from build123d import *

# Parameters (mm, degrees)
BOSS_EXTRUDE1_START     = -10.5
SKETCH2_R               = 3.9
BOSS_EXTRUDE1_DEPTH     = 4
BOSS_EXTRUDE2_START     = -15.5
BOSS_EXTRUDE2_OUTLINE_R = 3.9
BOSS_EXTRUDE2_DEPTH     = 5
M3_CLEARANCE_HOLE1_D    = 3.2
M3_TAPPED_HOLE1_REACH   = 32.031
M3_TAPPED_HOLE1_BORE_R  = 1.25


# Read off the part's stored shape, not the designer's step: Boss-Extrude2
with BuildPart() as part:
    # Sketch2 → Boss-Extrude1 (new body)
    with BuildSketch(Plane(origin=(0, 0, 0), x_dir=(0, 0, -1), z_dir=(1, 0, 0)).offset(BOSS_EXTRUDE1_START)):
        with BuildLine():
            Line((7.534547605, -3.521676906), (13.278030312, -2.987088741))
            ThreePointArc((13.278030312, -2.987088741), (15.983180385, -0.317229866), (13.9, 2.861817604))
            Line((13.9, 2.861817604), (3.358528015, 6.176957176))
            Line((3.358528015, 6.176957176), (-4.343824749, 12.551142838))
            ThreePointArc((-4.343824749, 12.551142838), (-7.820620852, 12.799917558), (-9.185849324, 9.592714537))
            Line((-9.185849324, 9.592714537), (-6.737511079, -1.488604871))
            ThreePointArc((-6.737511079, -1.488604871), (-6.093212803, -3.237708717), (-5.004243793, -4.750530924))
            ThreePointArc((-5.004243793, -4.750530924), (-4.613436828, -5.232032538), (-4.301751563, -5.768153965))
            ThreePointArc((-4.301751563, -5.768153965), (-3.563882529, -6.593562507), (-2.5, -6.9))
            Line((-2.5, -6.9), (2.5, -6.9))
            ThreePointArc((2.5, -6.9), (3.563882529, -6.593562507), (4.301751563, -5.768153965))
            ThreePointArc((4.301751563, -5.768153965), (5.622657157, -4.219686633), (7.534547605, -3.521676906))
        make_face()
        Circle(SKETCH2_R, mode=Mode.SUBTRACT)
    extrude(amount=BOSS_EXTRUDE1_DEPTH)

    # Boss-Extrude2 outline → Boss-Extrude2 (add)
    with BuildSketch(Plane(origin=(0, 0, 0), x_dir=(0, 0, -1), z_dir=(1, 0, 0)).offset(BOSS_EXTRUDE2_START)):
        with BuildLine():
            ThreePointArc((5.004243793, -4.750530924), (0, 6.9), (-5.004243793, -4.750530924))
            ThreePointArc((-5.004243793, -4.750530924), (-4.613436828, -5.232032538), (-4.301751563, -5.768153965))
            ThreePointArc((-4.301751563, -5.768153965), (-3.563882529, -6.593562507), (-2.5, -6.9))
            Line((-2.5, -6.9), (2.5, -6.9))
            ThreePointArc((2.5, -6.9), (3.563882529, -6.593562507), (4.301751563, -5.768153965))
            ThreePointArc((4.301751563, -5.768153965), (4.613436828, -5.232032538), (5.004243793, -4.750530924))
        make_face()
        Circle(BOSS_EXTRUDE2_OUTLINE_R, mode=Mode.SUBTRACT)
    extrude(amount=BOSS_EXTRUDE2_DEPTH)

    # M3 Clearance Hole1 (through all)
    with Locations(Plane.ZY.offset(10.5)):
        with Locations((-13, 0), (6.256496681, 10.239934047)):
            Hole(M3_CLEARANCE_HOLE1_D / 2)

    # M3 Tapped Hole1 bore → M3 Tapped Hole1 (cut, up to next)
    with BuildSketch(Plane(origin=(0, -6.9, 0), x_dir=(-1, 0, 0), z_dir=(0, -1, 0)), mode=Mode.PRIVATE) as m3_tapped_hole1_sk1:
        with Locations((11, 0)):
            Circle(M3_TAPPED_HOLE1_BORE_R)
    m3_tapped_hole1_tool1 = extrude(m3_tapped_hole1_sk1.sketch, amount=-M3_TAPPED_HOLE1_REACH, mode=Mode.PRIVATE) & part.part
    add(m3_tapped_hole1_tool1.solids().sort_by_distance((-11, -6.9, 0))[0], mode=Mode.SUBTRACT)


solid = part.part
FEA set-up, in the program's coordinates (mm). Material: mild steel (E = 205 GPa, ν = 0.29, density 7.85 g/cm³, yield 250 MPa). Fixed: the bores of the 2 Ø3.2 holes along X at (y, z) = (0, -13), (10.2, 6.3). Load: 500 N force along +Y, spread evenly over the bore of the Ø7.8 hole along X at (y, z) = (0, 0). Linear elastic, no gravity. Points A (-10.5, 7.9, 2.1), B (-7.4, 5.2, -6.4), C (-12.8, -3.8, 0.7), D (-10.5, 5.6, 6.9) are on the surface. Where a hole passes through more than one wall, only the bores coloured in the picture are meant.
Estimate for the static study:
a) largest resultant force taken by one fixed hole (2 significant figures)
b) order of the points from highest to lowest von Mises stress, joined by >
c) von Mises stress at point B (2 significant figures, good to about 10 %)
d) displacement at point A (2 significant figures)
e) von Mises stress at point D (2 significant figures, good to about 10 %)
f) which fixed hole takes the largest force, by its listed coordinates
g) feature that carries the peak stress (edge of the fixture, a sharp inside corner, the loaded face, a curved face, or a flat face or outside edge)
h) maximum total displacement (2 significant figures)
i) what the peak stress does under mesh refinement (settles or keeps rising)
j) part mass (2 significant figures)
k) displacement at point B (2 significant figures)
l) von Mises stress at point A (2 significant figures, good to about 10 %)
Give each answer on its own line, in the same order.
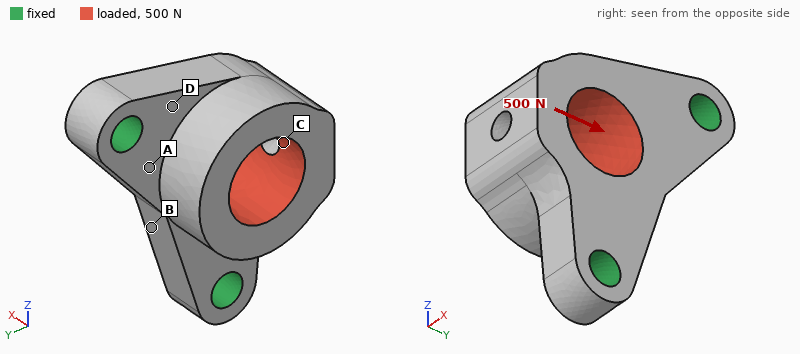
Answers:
370 N
D > A > B > C
11 MPa
0.95 µm
37 MPa
(10.2, 6.3)
edge of the fixture
6.2 µm
keeps rising
11 g
0.97 µm
31 MPa
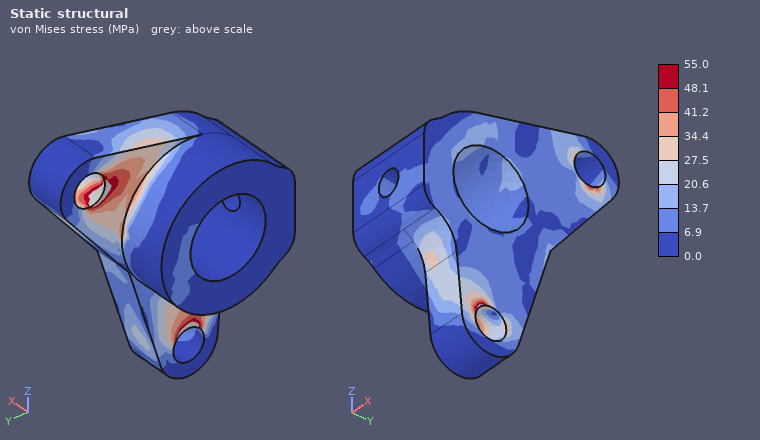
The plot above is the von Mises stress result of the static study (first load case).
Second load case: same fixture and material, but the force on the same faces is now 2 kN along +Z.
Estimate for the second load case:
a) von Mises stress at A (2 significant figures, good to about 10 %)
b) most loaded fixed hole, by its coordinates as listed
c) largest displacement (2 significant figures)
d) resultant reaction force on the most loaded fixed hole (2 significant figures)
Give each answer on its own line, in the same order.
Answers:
75 MPa
(0, -13)
14 µm
1.4 kN
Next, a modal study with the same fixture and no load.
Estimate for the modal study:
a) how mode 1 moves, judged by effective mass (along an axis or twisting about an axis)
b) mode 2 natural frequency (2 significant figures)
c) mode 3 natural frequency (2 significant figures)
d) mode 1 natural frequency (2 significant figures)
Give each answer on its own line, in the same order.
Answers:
along X
35 kHz
39 kHz
13 kHz
